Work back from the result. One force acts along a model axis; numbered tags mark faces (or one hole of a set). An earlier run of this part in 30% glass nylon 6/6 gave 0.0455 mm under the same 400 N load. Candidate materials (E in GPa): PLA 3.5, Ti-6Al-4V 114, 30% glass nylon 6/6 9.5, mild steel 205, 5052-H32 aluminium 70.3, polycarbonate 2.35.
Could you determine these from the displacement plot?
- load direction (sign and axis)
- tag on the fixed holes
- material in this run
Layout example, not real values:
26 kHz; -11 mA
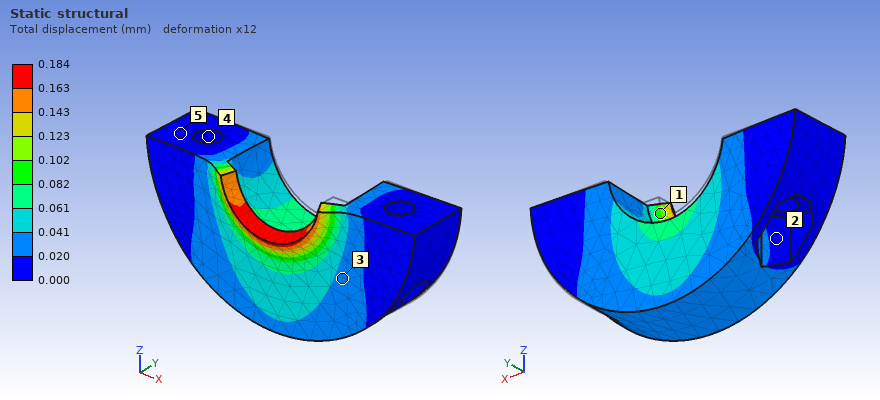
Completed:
-Y; 4; polycarbonate
